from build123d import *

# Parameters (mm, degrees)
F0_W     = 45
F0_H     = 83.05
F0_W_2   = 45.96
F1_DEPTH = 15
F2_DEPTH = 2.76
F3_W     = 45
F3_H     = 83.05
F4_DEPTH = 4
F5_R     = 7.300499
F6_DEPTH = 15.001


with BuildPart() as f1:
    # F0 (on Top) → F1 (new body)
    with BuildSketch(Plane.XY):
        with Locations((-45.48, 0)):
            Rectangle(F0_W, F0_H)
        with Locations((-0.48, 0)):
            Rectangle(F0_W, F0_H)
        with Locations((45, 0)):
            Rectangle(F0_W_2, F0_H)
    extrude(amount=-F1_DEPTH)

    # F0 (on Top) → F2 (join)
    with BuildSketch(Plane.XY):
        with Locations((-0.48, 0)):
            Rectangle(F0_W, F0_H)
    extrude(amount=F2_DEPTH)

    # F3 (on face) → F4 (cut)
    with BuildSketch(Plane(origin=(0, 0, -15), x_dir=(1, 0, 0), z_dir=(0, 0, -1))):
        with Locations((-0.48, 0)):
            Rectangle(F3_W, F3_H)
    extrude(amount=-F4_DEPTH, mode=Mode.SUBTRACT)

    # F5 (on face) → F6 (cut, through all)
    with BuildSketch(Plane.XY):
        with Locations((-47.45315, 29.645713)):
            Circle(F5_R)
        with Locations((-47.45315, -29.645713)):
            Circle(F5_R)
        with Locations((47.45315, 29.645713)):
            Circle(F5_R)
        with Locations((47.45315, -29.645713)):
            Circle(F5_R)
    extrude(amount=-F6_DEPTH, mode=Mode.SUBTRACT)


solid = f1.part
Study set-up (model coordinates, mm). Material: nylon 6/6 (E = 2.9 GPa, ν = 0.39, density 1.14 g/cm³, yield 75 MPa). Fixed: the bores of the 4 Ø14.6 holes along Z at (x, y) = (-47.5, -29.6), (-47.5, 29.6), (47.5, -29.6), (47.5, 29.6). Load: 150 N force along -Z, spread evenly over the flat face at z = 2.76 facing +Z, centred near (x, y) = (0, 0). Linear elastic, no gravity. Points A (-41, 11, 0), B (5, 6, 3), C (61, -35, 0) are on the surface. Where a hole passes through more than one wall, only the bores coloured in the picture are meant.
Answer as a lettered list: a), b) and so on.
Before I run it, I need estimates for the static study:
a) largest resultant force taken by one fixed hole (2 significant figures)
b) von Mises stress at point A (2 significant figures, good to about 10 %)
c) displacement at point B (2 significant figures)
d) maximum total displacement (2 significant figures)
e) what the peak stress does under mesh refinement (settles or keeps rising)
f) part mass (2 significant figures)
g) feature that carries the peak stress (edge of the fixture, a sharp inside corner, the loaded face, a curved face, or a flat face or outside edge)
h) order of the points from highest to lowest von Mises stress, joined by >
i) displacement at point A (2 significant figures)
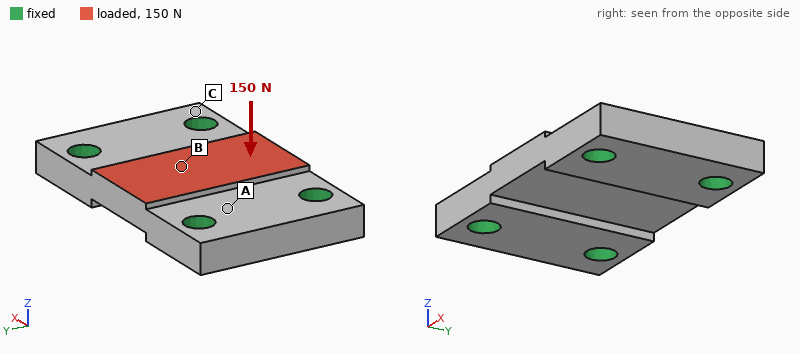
a) 48 N
b) 0.13 MPa
c) 8.6 µm
d) 9.0 µm
e) keeps rising
f) 180 g
g) edge of the fixture
h) B > A > C
i) 1.6 µm
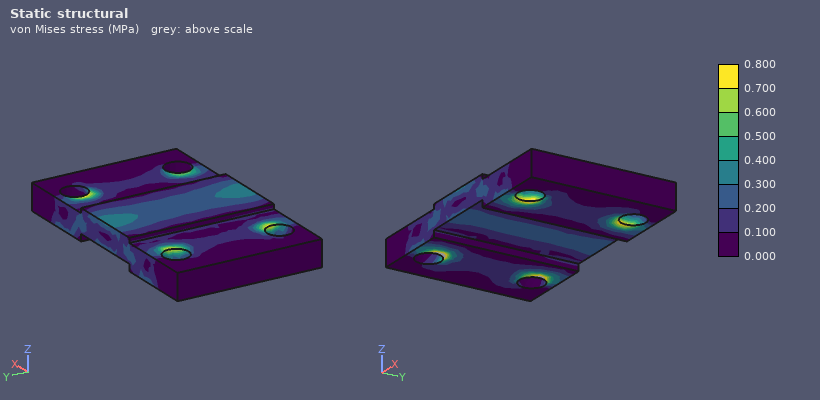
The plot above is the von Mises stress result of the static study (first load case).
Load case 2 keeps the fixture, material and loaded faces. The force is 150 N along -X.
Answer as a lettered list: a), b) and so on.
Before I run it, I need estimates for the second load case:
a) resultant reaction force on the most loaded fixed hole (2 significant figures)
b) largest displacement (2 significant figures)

a) 40 N
b) 1.3 µm
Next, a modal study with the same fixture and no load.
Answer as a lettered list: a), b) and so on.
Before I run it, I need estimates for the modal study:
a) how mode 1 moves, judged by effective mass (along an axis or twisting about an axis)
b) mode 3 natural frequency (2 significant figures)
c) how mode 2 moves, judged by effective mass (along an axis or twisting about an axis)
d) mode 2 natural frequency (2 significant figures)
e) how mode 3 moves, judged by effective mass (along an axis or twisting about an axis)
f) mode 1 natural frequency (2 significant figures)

a) along Z
b) 4900 Hz
c) twisting about X
d) 3400 Hz
e) along Y
f) 2700 Hz
